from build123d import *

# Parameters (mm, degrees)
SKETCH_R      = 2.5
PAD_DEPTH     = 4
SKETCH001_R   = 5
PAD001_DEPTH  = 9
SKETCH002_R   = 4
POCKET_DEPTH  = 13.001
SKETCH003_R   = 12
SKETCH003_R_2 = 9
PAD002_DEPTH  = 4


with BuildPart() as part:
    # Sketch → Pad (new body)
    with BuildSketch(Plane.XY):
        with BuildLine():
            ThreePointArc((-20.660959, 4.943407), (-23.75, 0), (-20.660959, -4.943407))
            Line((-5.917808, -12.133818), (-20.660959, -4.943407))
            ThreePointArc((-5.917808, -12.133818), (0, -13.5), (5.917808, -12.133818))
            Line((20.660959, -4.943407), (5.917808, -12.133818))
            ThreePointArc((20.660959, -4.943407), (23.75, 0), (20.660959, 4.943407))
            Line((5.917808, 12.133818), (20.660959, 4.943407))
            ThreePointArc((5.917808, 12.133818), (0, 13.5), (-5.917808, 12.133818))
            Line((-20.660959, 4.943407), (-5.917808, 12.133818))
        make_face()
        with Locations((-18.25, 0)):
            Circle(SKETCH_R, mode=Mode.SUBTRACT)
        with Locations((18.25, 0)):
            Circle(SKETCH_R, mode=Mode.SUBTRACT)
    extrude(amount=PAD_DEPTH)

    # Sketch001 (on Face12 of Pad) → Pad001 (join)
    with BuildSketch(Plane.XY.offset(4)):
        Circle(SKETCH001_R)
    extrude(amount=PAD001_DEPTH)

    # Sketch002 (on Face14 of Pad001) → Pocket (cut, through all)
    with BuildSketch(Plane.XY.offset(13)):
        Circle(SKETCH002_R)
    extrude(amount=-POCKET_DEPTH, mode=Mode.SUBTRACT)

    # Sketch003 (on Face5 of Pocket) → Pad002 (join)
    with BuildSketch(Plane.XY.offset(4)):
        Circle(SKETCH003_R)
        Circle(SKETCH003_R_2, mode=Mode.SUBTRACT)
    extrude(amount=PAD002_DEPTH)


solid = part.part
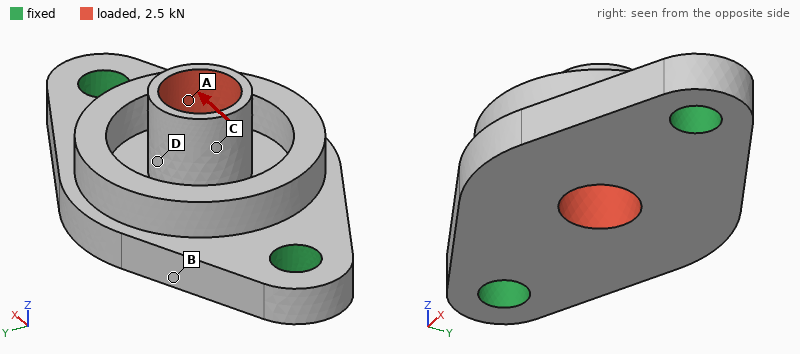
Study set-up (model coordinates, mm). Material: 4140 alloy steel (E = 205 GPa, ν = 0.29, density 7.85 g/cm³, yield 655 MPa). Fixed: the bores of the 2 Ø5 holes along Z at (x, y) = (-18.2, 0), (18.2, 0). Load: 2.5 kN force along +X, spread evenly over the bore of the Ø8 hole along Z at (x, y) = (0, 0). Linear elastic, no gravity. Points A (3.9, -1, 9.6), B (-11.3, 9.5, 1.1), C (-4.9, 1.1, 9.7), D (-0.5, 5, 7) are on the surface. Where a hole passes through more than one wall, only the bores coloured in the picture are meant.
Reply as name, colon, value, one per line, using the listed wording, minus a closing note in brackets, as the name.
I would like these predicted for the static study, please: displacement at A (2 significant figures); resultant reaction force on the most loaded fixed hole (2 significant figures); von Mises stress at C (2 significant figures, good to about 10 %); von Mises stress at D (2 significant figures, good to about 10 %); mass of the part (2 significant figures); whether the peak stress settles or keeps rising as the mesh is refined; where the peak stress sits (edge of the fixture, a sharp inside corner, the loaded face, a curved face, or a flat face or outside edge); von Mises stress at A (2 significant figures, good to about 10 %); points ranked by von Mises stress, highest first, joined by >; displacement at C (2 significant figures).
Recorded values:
displacement at A: 16 µm
resultant reaction force on the most loaded fixed hole: 1.3 kN
von Mises stress at C: 41 MPa
von Mises stress at D: 120 MPa
mass of the part: 32 g
whether the peak stress settles or keeps rising as the mesh is refined: keeps rising
where the peak stress sits: a sharp inside corner
von Mises stress at A: 61 MPa
points ranked by von Mises stress, highest first, joined by >: D > A > C > B
displacement at C: 17 µm
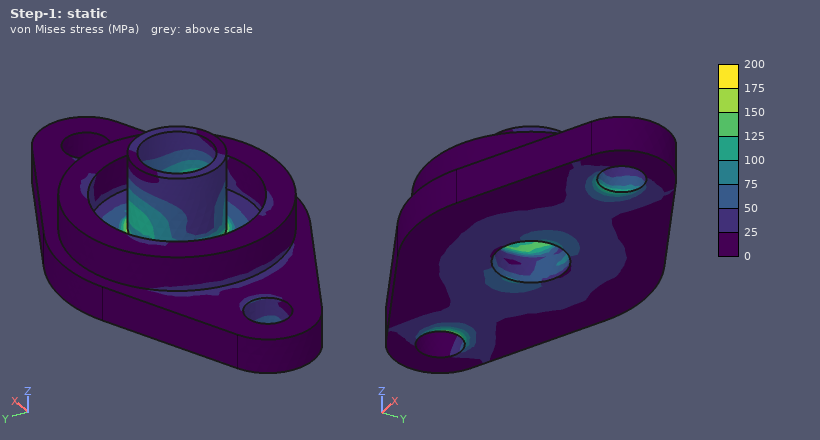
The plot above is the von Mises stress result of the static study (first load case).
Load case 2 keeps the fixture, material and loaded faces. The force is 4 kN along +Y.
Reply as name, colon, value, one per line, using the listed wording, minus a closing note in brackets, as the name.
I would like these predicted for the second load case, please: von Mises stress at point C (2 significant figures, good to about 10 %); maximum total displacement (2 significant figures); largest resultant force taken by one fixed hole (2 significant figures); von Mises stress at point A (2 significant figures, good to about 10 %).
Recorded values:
von Mises stress at point C: 120 MPa
maximum total displacement: 68 µm
largest resultant force taken by one fixed hole: 2.0 kN
von Mises stress at point A: 150 MPa
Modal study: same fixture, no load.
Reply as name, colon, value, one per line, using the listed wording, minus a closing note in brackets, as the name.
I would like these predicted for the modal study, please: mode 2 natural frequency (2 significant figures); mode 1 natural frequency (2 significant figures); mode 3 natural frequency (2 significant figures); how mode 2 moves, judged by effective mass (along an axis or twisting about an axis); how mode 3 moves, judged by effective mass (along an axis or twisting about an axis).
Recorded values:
mode 2 natural frequency: 13 kHz
mode 1 natural frequency: 11 kHz
mode 3 natural frequency: 29 kHz
how mode 2 moves, judged by effective mass: along Z
how mode 3 moves, judged by effective mass: along Y
